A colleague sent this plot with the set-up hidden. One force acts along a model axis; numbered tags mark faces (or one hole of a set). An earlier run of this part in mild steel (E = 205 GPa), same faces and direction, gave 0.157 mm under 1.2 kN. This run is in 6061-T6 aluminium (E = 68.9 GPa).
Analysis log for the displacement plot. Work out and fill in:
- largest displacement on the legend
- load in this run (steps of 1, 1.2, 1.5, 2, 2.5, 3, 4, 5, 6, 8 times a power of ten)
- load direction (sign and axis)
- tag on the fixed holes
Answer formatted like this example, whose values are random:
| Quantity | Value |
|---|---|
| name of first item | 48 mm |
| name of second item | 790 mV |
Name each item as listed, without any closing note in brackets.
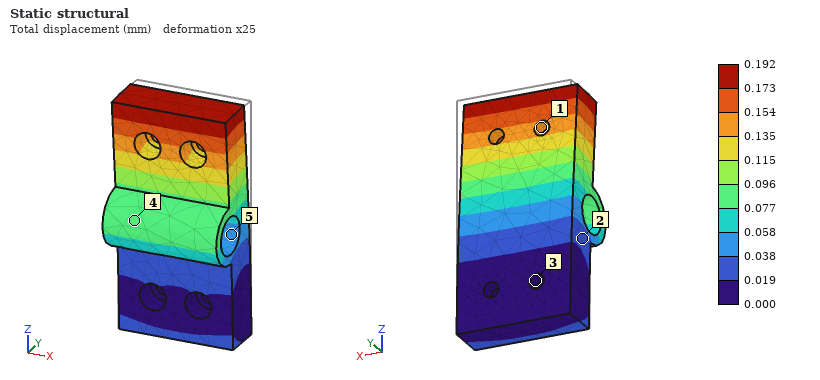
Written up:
| Quantity | Value |
|---|---|
| largest displacement on the legend | 0.192 mm |
| load in this run | 500 N |
| load direction | -Y |
| tag on the fixed holes | 3 |
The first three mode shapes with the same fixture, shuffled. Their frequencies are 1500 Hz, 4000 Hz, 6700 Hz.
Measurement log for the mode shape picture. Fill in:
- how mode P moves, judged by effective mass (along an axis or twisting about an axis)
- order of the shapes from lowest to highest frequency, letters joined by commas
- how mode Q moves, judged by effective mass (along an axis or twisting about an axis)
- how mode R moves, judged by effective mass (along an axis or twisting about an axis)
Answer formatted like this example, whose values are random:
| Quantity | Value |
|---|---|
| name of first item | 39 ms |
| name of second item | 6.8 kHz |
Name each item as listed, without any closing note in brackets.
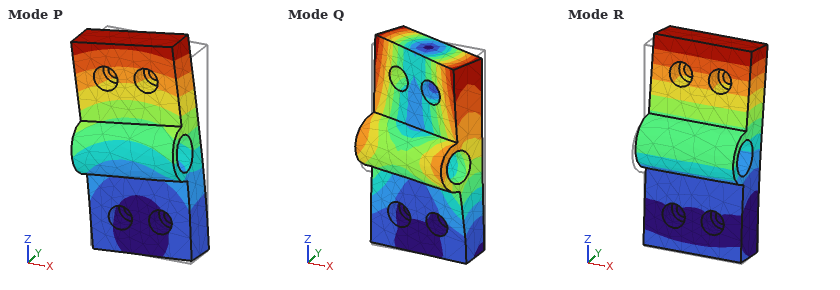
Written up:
| Quantity | Value |
|---|---|
| how mode P moves, judged by effective mass | along X |
| order of the shapes from lowest to highest frequency, letters joined by commas | R, P, Q |
| how mode Q moves, judged by effective mass | twisting about Z |
| how mode R moves, judged by effective mass | along Y |
